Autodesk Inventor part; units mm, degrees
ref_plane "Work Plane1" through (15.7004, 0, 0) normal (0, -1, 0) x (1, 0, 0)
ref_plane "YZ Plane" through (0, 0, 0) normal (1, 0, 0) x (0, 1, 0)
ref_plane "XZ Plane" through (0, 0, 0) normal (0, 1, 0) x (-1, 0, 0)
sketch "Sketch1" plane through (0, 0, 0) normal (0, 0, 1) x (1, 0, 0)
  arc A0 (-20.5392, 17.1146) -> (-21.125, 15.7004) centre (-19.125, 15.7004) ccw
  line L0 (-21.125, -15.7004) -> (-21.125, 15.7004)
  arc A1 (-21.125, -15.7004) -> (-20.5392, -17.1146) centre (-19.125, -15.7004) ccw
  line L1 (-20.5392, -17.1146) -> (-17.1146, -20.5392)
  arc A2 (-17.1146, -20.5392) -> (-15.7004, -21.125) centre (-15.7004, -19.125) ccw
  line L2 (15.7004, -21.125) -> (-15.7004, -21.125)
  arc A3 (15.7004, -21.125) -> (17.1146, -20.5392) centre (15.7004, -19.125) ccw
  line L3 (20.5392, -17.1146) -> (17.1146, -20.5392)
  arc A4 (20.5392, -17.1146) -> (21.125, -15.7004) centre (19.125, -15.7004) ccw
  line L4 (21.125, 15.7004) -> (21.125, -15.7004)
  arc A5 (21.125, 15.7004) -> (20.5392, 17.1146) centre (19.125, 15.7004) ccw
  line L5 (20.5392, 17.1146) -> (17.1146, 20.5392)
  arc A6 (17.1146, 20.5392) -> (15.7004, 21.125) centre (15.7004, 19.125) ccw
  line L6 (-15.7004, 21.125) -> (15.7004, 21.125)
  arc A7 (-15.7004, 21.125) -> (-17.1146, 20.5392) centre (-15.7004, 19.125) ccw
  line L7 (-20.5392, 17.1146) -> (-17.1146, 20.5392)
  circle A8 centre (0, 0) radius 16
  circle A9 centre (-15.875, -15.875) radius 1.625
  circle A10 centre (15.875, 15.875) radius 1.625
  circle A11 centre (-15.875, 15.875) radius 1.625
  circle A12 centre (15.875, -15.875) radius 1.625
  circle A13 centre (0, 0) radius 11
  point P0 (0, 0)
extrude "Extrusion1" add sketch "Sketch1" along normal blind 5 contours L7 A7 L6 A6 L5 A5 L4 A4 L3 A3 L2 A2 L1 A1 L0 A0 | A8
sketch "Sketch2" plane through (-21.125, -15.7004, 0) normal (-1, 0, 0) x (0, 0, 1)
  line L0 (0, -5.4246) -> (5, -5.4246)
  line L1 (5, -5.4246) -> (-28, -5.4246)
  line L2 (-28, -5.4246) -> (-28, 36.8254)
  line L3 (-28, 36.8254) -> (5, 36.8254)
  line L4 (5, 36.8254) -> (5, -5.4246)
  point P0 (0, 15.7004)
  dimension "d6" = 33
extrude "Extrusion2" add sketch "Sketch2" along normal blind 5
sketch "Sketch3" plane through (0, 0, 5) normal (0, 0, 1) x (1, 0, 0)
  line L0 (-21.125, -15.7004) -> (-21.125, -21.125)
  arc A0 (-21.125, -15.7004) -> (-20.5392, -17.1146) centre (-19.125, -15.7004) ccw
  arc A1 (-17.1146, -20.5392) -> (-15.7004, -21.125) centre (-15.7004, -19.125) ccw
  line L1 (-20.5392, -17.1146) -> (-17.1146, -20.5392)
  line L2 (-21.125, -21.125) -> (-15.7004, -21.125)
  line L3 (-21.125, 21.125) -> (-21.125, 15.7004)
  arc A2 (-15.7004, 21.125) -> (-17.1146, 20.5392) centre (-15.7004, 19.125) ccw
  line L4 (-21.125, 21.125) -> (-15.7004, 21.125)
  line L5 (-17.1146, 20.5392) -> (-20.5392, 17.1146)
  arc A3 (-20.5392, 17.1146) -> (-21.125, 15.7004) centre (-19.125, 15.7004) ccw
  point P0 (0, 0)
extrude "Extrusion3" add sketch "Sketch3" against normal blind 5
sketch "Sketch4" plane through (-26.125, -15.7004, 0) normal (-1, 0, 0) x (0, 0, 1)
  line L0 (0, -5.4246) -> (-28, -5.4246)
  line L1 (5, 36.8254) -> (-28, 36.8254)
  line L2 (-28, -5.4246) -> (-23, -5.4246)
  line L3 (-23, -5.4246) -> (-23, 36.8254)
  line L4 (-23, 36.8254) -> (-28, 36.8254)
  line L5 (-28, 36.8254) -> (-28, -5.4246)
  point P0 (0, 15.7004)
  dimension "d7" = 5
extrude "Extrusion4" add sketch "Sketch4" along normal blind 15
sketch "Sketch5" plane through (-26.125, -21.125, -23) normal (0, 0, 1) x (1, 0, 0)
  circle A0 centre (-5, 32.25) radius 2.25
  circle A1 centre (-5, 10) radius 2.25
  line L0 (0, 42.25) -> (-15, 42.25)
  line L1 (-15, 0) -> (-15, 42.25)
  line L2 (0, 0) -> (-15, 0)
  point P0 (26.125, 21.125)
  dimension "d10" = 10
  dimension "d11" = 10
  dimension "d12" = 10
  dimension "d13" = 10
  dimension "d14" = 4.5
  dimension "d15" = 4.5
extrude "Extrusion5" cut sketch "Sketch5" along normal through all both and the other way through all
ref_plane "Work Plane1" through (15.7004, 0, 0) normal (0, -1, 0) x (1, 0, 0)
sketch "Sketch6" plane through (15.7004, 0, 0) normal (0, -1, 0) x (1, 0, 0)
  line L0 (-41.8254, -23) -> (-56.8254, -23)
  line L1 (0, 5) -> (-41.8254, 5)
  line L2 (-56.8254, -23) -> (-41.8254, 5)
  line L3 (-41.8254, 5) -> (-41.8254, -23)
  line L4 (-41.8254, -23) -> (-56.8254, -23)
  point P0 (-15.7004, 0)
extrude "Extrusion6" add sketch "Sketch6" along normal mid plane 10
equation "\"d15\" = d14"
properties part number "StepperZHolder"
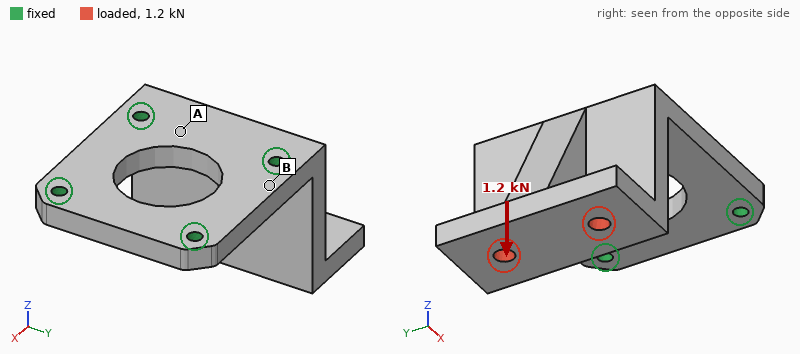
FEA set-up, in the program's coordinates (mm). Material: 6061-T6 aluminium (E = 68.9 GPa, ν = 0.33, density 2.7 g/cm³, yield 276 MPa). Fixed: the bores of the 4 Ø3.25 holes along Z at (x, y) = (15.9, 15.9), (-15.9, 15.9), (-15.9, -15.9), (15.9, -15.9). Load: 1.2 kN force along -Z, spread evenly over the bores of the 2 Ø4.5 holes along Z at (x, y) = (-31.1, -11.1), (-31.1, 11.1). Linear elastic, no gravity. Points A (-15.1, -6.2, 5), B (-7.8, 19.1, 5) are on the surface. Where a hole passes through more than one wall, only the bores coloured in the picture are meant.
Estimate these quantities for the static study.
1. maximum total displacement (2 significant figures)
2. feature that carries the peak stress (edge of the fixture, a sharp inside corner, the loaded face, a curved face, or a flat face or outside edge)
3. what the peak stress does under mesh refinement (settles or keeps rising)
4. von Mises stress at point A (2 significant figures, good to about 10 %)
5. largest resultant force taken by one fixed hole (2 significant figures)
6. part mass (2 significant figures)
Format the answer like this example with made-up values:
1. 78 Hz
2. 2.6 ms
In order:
1. 0.23 mm
2. edge of the fixture
3. keeps rising
4. 42 MPa
5. 660 N
6. 51 g
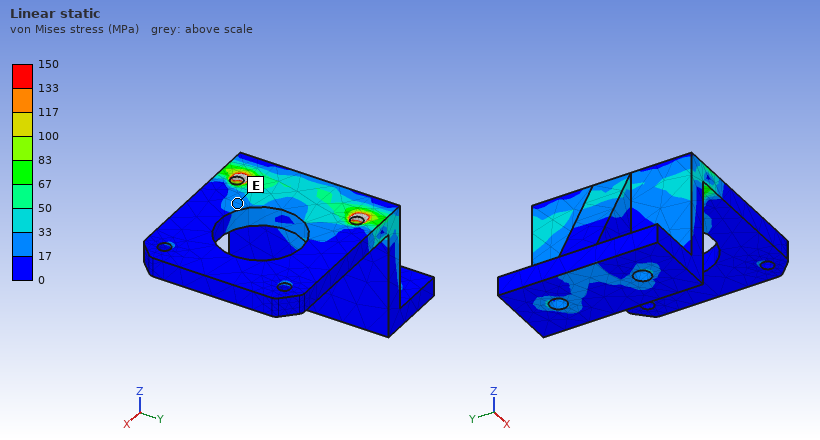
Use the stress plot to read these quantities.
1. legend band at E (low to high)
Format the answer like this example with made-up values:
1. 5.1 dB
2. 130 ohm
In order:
1. 17 to 33 MPa
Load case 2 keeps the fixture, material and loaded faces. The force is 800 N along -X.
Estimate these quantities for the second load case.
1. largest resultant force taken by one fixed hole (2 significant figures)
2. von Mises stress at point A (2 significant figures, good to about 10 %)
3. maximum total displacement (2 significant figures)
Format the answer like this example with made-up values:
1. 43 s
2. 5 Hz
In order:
1. 390 N
2. 62 MPa
3. 0.37 mm
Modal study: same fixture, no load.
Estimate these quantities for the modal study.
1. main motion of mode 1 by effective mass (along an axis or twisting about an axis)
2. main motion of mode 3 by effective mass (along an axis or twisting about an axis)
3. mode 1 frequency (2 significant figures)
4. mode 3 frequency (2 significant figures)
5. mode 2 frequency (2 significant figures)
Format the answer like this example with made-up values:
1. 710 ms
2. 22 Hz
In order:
1. along X
2. along Y
3. 1900 Hz
4. 6900 Hz
5. 6200 Hz
